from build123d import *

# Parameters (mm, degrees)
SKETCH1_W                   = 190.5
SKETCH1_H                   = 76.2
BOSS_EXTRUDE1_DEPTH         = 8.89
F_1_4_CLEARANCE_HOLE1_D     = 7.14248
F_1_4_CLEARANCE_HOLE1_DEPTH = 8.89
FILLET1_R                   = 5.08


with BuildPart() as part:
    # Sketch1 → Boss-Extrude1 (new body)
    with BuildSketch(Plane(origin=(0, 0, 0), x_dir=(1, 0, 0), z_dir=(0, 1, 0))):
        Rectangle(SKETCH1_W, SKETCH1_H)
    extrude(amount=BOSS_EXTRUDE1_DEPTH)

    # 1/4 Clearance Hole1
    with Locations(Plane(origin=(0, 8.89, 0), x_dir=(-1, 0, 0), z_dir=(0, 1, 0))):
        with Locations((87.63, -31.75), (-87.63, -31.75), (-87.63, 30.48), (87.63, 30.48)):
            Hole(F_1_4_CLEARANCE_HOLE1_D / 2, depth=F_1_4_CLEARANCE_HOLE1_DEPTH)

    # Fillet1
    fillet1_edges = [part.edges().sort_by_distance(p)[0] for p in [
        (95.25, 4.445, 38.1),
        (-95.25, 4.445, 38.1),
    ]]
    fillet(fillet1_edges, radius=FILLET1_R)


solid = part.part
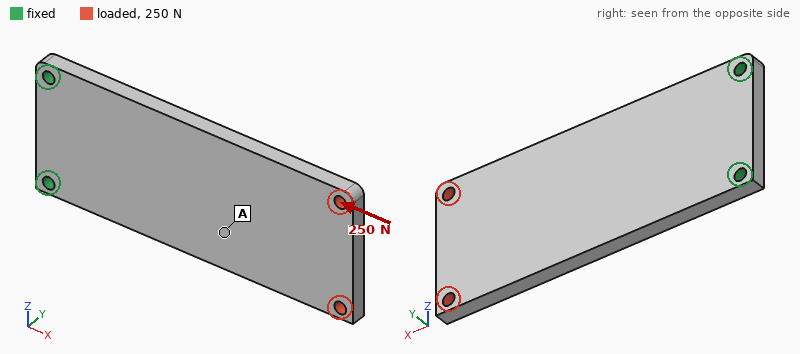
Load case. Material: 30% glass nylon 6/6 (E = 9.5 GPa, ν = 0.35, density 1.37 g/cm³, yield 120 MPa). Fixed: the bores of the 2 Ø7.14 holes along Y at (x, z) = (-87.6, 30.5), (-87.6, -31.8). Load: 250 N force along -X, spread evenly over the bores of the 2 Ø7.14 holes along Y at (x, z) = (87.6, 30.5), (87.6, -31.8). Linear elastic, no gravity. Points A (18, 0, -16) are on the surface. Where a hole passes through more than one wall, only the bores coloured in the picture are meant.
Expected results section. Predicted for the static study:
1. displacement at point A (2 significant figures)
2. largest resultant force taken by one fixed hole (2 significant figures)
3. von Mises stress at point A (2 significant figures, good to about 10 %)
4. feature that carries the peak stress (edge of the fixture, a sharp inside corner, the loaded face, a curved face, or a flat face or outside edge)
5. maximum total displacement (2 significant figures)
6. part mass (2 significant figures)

5.0 µm
130 N
0.37 MPa
the loaded face
11 µm
170 g
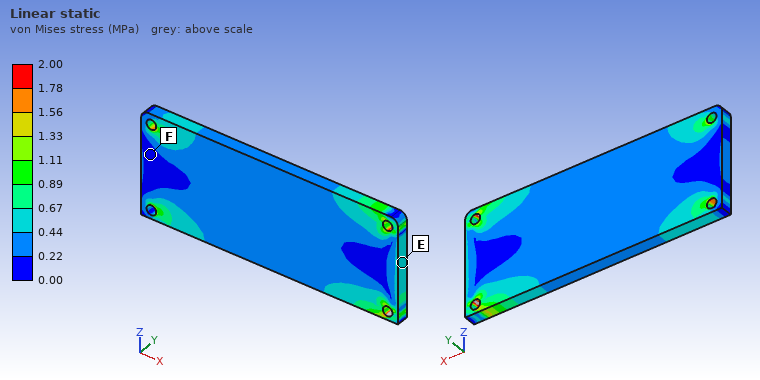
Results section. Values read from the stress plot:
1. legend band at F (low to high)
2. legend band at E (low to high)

0.00 to 0.22 MPa
0.44 to 0.67 MPa
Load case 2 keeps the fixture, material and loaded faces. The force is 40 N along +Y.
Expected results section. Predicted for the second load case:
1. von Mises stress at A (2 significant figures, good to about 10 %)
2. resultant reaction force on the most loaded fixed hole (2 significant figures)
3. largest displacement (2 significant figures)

2.8 MPa
21 N
2.0 mm
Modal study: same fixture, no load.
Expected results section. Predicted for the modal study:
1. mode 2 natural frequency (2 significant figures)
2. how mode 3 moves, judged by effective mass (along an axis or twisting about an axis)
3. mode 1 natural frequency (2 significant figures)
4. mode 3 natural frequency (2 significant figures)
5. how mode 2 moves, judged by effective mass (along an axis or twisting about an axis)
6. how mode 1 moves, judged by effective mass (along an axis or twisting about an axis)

560 Hz
along Y
110 Hz
680 Hz
twisting about X
along Y
